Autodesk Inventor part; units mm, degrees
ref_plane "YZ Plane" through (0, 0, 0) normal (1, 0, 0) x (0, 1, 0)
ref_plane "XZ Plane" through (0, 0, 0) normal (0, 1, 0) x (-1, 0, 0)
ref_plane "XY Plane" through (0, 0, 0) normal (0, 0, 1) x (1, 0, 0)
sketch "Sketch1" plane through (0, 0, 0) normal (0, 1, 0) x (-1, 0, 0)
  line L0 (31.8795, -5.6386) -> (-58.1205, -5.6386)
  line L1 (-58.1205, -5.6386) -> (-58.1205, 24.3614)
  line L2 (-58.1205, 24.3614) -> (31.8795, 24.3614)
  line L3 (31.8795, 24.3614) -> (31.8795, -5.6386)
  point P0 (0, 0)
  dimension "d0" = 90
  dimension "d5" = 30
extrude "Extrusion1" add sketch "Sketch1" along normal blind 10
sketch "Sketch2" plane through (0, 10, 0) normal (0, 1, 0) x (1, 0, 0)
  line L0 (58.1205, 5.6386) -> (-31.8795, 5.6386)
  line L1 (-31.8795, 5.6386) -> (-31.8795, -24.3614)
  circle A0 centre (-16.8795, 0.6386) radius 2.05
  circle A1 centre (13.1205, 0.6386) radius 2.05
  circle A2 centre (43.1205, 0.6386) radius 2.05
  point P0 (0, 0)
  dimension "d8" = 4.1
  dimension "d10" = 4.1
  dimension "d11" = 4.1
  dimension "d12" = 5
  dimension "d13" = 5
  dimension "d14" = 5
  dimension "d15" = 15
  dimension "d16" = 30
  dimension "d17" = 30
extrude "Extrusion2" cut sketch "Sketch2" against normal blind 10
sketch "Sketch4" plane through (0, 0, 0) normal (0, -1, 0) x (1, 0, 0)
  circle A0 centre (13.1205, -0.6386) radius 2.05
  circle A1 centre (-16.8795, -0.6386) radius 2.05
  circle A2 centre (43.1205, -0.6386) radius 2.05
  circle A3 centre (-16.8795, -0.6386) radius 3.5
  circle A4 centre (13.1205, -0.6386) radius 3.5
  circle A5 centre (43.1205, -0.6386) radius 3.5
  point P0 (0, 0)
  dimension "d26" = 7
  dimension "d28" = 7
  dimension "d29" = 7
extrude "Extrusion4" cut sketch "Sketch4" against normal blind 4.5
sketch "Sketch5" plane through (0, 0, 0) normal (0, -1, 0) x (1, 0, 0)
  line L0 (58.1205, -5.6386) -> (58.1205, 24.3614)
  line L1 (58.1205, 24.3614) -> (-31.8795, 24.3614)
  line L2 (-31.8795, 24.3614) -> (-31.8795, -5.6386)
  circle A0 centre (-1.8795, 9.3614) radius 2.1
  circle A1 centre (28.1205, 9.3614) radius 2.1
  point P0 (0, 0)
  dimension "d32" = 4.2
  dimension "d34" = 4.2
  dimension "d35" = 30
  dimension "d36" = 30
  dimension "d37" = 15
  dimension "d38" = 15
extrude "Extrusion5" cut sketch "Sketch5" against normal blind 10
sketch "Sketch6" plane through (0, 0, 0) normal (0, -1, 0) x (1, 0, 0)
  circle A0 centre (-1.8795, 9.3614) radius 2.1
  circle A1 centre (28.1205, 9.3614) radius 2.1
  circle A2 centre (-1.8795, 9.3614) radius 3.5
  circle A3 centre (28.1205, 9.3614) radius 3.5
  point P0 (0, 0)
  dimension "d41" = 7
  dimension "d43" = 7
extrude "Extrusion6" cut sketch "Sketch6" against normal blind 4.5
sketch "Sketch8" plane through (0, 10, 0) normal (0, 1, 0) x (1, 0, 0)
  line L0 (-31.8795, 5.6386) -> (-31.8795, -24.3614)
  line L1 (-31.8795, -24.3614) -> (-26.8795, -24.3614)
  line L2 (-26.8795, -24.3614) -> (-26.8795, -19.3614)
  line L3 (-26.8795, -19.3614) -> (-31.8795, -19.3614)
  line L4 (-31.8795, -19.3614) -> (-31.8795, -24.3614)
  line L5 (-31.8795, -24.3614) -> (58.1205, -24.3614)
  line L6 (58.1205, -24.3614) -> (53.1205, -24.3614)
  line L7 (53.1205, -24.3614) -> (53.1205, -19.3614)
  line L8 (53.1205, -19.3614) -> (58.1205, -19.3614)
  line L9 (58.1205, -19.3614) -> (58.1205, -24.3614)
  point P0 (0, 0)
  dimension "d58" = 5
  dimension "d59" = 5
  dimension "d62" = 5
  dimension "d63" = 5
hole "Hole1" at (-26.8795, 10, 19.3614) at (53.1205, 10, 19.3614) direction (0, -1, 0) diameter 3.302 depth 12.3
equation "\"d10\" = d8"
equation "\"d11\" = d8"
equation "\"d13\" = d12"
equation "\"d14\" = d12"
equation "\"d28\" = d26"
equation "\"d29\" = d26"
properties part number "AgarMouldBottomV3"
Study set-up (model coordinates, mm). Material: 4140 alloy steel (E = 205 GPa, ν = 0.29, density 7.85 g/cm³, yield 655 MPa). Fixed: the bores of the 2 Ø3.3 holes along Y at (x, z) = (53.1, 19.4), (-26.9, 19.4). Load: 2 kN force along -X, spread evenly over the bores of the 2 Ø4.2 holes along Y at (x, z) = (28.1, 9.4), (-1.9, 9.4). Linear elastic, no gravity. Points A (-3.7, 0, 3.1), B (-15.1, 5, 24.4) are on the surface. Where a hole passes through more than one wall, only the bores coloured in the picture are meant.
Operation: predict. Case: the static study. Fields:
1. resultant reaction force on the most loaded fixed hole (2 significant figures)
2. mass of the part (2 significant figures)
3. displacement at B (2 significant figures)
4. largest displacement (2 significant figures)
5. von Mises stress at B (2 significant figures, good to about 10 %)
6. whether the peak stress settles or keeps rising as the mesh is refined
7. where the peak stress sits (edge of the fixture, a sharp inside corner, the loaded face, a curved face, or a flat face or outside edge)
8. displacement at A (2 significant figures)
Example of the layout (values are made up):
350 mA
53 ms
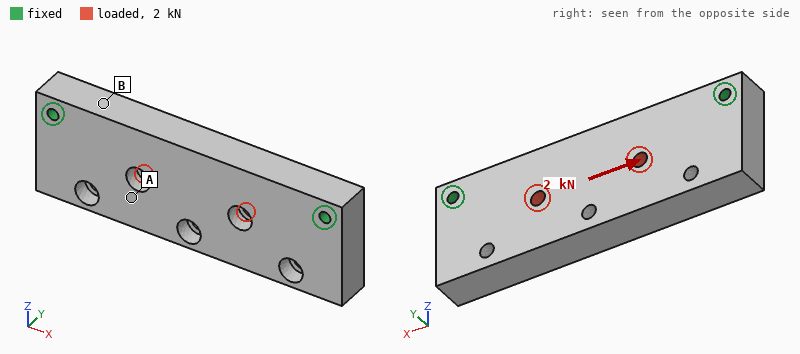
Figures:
1.0 kN
200 g
0.40 µm
1.4 µm
7.1 MPa
keeps rising
edge of the fixture
0.92 µm
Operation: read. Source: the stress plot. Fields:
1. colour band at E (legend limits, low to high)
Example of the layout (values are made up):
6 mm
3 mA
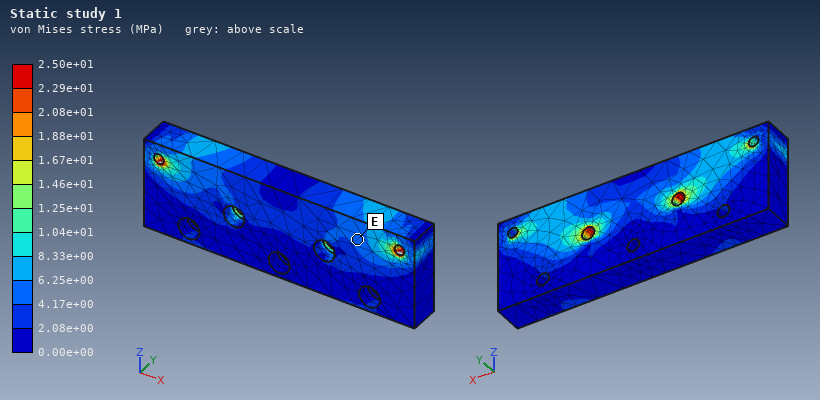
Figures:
4.17e+00 to 6.25e+00 MPa
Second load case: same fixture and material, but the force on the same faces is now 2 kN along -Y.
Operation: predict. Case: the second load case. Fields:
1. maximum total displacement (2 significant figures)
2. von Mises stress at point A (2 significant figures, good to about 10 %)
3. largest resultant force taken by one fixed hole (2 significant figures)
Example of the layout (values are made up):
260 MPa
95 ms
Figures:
24 µm
22 MPa
1.0 kN
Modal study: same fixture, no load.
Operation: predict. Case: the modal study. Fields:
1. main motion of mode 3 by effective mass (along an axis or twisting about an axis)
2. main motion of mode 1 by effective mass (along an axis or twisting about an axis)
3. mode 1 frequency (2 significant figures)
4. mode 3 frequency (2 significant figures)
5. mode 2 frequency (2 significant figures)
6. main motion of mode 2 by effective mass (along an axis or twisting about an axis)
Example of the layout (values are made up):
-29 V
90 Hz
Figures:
along Z
along Y
4800 Hz
11 kHz
8900 Hz
twisting about X
